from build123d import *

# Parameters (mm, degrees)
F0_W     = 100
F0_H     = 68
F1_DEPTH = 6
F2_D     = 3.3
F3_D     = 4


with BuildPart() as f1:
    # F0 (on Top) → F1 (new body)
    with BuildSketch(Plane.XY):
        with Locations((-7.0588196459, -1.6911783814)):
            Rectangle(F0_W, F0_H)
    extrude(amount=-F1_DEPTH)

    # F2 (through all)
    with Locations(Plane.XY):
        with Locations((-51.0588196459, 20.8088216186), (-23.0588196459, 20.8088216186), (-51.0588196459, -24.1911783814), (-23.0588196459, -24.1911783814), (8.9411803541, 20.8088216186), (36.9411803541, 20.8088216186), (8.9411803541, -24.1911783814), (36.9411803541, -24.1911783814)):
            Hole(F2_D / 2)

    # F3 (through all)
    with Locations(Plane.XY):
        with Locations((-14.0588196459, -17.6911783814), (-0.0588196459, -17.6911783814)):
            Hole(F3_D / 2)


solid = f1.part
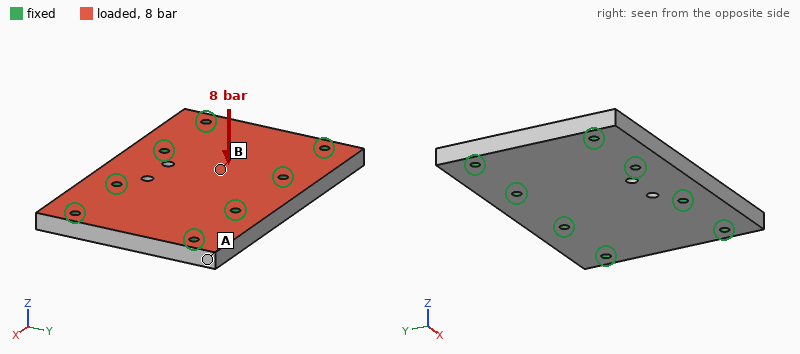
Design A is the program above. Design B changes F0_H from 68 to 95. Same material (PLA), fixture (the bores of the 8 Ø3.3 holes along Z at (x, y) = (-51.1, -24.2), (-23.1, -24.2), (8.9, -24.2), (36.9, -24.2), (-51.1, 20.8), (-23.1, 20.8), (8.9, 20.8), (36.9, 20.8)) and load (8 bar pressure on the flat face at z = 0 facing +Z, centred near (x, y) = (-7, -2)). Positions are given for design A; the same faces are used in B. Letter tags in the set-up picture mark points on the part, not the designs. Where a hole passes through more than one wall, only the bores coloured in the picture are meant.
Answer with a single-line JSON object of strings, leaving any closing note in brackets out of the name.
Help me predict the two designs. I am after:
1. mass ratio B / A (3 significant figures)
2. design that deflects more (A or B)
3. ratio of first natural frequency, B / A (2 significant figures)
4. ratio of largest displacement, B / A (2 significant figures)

{"mass ratio B / A": "1.40", "design that deflects more": "B", "ratio of first natural frequency, B / A": "0.56", "ratio of largest displacement, B / A": "3.4"}
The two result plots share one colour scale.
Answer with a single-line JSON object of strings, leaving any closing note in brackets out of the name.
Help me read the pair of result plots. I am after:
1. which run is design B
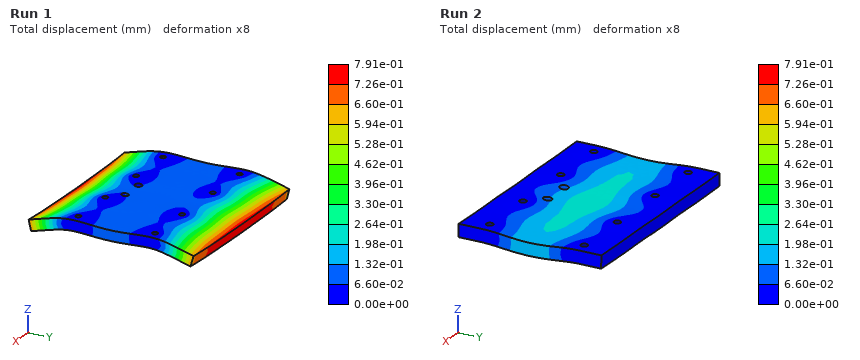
{"which run is design B": "Run 1"}
